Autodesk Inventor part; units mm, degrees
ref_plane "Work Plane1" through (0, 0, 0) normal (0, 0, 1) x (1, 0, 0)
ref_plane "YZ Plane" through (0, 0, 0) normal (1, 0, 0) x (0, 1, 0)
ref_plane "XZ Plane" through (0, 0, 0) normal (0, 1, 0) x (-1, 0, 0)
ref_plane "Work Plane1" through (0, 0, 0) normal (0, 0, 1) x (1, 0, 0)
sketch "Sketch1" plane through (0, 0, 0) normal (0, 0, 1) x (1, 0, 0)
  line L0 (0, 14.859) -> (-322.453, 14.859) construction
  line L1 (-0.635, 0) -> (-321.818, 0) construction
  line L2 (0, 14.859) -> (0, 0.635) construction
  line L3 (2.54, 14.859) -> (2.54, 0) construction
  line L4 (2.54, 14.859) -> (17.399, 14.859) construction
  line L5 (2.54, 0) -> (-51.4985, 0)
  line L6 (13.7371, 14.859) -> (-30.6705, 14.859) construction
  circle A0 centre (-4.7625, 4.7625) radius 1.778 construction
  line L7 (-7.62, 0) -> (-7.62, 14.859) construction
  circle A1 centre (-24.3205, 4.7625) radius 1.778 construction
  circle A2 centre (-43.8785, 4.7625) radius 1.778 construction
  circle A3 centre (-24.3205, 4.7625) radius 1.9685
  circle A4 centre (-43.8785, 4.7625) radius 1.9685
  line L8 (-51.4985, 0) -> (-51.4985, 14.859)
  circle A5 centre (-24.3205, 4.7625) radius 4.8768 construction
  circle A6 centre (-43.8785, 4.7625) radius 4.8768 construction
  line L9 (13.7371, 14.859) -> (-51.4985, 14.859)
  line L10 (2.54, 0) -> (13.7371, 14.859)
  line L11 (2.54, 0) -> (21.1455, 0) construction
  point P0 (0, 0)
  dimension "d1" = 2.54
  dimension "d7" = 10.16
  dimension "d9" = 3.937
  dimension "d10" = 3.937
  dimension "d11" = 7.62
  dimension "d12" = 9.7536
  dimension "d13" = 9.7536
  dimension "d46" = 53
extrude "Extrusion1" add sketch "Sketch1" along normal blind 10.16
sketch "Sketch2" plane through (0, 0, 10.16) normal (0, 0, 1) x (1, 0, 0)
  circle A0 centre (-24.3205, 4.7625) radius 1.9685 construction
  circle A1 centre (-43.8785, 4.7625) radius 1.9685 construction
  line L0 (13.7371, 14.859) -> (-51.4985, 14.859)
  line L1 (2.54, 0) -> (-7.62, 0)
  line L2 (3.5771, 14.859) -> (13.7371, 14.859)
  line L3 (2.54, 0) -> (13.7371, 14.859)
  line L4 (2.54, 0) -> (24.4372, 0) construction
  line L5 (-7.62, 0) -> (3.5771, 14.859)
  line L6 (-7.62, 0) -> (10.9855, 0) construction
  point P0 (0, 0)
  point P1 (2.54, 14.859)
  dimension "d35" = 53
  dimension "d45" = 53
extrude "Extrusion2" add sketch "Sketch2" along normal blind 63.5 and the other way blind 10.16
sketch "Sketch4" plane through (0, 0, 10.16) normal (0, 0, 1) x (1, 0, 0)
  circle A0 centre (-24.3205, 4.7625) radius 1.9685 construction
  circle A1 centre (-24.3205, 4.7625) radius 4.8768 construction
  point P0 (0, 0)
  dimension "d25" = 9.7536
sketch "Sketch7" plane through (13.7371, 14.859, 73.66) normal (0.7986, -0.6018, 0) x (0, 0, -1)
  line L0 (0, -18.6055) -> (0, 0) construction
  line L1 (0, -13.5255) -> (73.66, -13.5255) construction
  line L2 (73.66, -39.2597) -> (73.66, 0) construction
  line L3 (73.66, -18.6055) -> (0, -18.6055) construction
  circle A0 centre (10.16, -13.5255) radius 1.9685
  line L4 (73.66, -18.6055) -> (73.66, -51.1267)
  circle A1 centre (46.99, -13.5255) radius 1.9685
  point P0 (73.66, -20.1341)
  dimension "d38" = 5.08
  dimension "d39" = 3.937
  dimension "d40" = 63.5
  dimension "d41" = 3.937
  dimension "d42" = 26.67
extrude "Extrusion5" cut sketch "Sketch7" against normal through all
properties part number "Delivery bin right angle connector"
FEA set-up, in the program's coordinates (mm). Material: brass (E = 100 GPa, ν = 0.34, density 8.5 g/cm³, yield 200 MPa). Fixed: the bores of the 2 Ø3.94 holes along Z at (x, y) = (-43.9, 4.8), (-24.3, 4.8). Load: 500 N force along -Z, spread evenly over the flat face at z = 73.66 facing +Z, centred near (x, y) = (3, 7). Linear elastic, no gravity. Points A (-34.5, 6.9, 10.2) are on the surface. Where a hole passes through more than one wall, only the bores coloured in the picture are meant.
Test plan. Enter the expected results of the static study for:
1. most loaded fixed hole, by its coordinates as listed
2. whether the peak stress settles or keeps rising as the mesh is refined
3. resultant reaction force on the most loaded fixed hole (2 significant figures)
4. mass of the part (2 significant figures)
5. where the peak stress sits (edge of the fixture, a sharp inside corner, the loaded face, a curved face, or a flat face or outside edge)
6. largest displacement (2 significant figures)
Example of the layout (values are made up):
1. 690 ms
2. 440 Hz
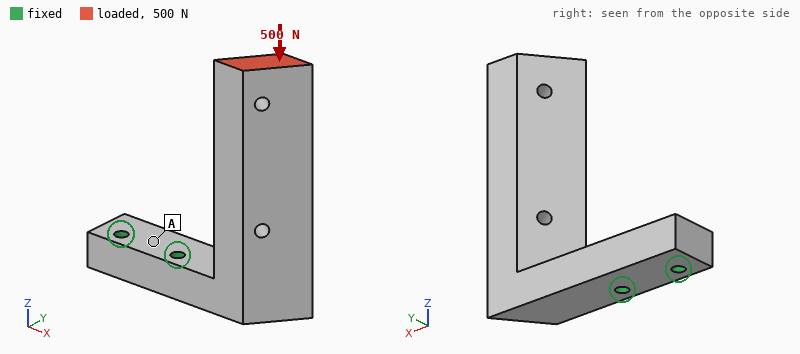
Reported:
1. (-24.3, 4.8)
2. keeps rising
3. 650 N
4. 150 g
5. edge of the fixture
6. 0.12 mm
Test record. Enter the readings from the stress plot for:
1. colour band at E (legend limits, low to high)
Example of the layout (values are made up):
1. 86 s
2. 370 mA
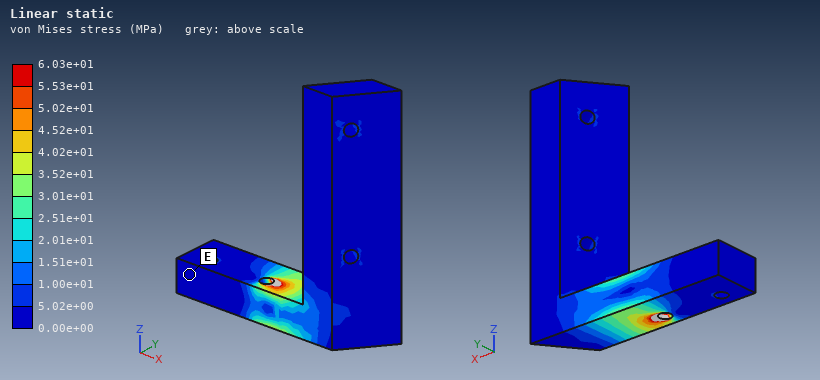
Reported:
1. 0.00e+00 to 5.02e+00 MPa
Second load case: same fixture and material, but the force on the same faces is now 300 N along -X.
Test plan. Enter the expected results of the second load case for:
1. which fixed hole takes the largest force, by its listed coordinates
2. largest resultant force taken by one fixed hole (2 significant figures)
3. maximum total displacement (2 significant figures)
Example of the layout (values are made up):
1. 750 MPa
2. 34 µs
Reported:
1. (-24.3, 4.8)
2. 350 N
3. 0.57 mm
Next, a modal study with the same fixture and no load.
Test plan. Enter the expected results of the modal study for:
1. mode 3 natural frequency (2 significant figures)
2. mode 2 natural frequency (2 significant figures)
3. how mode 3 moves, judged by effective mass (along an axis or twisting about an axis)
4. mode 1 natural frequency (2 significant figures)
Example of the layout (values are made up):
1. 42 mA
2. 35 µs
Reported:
1. 2800 Hz
2. 850 Hz
3. along Z
4. 660 Hz
